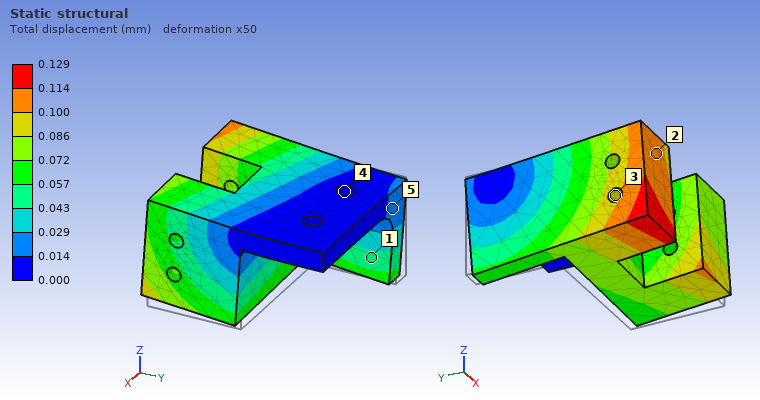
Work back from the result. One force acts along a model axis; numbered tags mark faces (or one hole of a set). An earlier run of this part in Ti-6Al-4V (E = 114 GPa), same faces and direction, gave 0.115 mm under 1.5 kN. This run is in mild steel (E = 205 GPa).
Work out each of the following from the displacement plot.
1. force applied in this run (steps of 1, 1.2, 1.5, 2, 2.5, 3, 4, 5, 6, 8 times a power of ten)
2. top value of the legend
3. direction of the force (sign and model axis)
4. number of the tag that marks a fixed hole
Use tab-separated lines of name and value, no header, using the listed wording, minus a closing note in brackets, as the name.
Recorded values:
force applied in this run	3 kN
top value of the legend	0.129 mm
direction of the force	+Z
number of the tag that marks a fixed hole	4
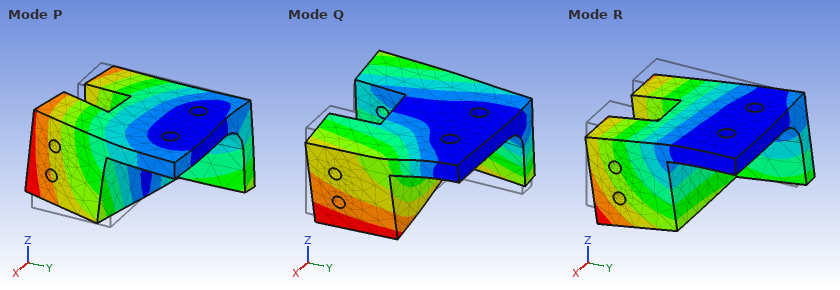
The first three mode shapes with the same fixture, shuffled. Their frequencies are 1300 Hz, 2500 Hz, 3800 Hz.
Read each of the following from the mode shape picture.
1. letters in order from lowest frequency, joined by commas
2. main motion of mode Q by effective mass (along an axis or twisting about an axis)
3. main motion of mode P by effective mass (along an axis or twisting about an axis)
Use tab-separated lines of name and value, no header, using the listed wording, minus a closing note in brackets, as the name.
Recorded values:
letters in order from lowest frequency, joined by commas	R, Q, P
main motion of mode Q by effective mass	along X
main motion of mode P by effective mass	along X
